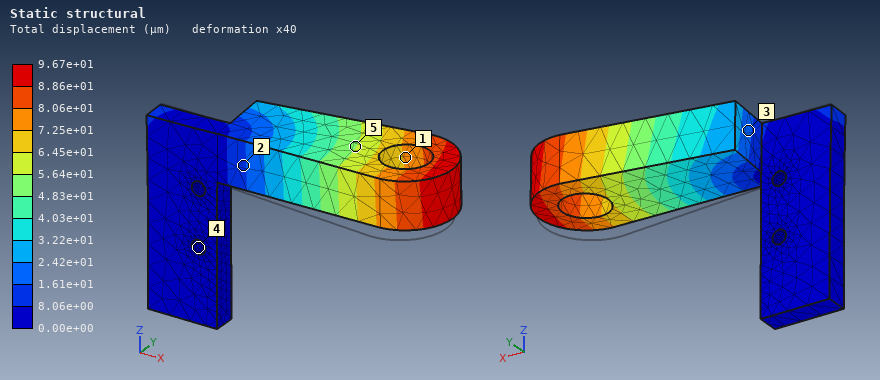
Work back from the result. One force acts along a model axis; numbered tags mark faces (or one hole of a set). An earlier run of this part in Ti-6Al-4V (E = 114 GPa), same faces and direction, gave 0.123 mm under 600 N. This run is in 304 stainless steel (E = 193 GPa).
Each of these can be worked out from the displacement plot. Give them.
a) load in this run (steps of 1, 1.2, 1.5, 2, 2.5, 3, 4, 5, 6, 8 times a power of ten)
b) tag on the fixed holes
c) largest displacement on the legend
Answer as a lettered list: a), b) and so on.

a) 800 N
b) 4
c) 9.67e+01 µm
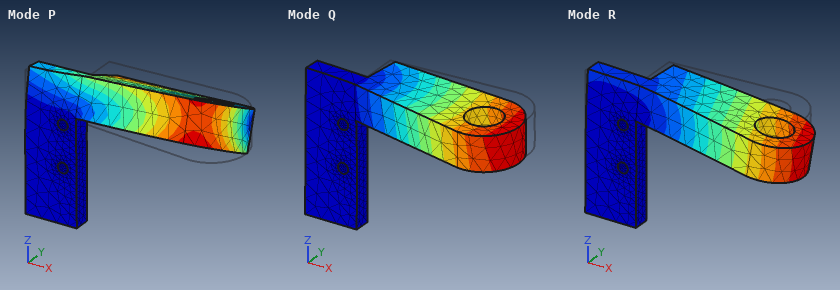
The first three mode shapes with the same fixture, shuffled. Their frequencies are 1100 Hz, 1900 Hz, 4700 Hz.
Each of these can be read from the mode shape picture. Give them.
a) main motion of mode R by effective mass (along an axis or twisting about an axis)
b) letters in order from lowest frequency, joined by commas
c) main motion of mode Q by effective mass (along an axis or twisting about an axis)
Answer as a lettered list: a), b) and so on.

a) along Z
b) Q, R, P
c) along Y
